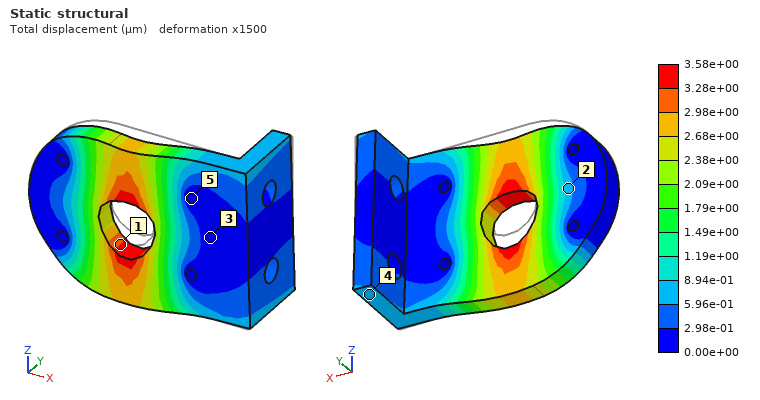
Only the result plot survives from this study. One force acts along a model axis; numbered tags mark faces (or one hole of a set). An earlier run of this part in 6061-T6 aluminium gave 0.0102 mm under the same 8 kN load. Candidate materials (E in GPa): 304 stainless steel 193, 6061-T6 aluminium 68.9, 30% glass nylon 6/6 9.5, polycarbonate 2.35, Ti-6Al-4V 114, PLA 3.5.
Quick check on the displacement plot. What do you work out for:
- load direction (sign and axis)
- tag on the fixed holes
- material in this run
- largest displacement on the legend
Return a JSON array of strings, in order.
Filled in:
["-Z", "5", "304 stainless steel", "3.58e+00 µm"]
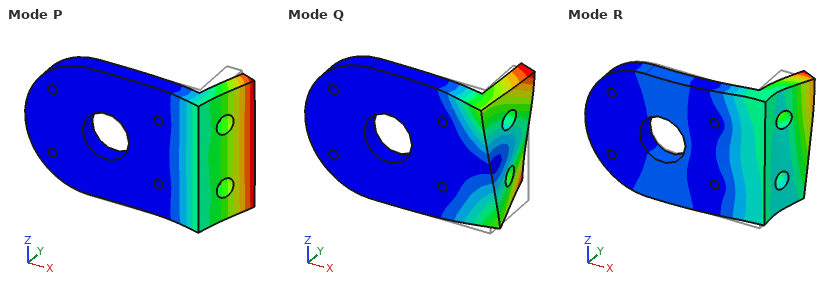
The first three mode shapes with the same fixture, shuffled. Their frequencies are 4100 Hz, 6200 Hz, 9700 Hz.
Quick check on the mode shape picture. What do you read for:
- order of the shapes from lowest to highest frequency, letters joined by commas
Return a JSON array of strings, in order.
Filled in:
["P, Q, R"]
